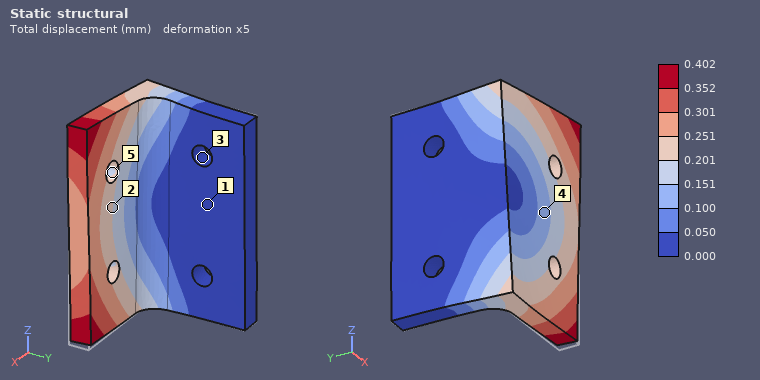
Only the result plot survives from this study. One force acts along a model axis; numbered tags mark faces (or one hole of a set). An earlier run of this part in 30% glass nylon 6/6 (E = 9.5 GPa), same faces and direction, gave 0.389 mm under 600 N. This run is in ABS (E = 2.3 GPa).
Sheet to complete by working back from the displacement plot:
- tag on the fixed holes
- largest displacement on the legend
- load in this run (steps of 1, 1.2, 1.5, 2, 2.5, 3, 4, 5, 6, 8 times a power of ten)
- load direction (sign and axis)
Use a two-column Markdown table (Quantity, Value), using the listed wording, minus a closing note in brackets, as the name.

| Quantity | Value |
|---|---|
| tag on the fixed holes | 3 |
| largest displacement on the legend | 0.402 mm |
| load in this run | 150 N |
| load direction | +Z |
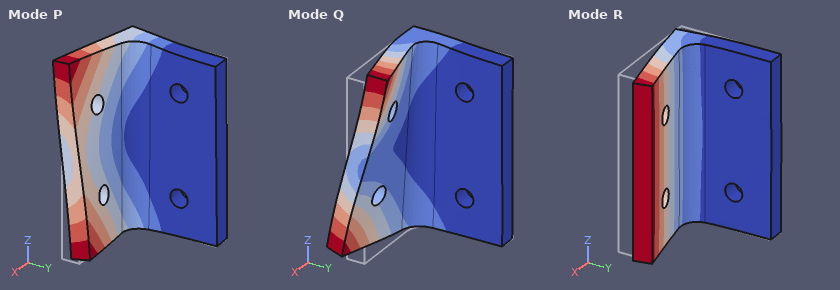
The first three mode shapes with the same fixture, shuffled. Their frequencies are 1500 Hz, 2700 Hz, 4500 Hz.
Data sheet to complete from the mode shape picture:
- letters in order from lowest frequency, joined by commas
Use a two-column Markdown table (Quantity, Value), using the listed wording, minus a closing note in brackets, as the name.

| Quantity | Value |
|---|---|
| letters in order from lowest frequency, joined by commas | R, P, Q |
